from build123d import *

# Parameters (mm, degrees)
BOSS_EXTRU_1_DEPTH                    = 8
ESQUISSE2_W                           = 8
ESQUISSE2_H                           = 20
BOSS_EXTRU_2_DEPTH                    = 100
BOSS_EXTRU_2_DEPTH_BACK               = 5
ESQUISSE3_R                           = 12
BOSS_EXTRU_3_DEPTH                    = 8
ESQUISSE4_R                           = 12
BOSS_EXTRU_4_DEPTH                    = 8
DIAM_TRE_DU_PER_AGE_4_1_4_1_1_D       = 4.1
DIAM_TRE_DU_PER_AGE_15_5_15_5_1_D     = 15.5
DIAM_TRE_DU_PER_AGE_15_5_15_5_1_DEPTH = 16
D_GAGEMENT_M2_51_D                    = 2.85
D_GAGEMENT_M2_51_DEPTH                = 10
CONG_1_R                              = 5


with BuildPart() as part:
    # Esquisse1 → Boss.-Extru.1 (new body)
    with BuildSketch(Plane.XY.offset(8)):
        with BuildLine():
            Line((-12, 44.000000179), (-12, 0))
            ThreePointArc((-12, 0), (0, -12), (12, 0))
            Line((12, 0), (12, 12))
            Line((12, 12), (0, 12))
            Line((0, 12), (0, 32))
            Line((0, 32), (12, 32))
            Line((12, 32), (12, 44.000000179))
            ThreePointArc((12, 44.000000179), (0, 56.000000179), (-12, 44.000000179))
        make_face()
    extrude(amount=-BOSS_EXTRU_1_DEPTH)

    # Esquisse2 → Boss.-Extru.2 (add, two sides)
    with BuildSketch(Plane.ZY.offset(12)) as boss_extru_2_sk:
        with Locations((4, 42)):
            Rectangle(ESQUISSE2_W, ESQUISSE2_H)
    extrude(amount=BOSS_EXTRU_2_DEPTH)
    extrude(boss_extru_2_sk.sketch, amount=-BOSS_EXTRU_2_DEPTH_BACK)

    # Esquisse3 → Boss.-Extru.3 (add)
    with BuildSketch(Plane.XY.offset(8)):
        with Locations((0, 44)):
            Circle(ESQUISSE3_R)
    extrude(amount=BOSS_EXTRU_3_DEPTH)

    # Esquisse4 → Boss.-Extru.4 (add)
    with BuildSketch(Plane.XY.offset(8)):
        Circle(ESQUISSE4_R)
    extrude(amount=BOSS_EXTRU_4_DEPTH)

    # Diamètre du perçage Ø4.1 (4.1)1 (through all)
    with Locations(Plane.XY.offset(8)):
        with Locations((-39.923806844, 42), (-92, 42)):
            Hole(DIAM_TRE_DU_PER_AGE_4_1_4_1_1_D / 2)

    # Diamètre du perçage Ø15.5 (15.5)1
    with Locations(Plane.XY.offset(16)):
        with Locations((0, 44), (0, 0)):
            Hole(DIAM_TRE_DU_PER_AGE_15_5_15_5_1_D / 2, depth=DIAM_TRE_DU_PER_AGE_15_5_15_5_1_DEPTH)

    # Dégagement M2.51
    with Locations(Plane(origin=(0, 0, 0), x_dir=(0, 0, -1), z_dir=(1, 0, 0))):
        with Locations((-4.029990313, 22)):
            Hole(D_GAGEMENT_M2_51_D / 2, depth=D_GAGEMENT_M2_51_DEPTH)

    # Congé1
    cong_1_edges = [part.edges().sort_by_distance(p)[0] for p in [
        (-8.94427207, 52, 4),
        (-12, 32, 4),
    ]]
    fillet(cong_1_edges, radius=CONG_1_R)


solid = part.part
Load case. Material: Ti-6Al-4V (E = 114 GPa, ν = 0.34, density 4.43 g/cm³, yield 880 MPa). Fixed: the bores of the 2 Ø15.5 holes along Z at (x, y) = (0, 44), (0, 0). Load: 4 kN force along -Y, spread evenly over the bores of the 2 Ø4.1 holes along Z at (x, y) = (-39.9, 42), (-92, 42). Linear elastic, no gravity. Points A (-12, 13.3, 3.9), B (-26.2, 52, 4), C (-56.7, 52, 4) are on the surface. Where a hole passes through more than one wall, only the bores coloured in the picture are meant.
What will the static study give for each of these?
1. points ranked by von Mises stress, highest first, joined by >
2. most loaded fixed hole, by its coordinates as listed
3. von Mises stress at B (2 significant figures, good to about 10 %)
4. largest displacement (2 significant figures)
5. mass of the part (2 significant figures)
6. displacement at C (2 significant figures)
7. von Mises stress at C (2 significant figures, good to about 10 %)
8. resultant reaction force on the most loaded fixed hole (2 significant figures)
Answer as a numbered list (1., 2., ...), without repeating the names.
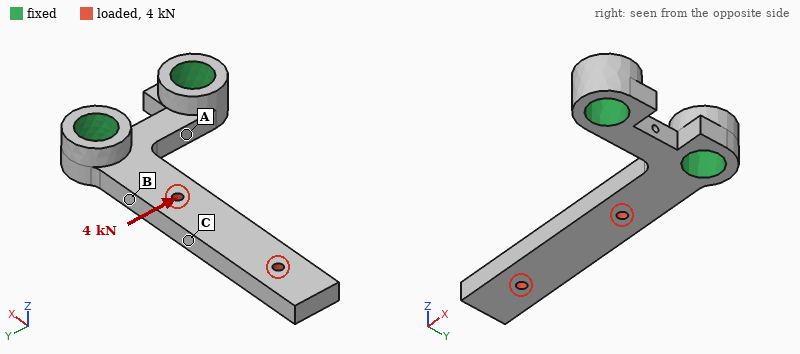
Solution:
1. B > C > A
2. (0, 0)
3. 300 MPa
4. 1.1 mm
5. 120 g
6. 0.39 mm
7. 130 MPa
8. 3.4 kN
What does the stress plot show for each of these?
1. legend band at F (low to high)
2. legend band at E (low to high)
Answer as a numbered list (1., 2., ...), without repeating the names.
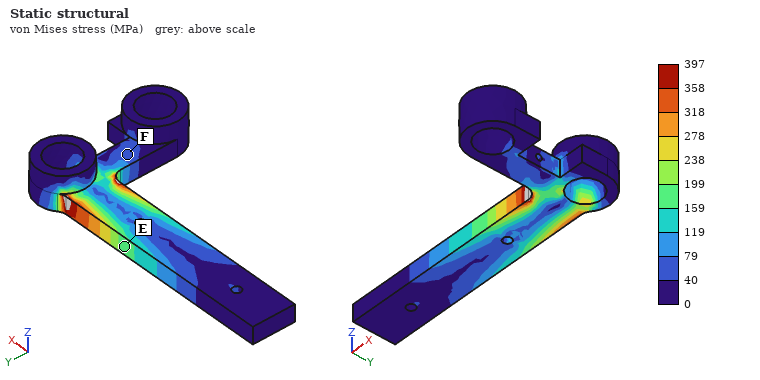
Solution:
1. 40 to 79 MPa
2. 159 to 199 MPa
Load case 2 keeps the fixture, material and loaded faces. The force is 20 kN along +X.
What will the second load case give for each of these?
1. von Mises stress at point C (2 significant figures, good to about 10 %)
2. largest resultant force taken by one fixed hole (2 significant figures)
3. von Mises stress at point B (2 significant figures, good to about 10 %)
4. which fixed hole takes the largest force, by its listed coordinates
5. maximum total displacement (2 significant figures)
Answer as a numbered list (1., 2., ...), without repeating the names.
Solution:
1. 66 MPa
2. 19 kN
3. 120 MPa
4. (0, 44)
5. 78 µm
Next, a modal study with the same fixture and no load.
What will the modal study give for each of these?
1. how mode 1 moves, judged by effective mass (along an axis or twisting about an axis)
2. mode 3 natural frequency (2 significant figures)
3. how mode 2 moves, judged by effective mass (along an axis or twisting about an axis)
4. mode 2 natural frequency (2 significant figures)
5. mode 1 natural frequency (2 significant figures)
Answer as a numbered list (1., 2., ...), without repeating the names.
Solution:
1. along Z
2. 3700 Hz
3. along Y
4. 1500 Hz
5. 610 Hz
